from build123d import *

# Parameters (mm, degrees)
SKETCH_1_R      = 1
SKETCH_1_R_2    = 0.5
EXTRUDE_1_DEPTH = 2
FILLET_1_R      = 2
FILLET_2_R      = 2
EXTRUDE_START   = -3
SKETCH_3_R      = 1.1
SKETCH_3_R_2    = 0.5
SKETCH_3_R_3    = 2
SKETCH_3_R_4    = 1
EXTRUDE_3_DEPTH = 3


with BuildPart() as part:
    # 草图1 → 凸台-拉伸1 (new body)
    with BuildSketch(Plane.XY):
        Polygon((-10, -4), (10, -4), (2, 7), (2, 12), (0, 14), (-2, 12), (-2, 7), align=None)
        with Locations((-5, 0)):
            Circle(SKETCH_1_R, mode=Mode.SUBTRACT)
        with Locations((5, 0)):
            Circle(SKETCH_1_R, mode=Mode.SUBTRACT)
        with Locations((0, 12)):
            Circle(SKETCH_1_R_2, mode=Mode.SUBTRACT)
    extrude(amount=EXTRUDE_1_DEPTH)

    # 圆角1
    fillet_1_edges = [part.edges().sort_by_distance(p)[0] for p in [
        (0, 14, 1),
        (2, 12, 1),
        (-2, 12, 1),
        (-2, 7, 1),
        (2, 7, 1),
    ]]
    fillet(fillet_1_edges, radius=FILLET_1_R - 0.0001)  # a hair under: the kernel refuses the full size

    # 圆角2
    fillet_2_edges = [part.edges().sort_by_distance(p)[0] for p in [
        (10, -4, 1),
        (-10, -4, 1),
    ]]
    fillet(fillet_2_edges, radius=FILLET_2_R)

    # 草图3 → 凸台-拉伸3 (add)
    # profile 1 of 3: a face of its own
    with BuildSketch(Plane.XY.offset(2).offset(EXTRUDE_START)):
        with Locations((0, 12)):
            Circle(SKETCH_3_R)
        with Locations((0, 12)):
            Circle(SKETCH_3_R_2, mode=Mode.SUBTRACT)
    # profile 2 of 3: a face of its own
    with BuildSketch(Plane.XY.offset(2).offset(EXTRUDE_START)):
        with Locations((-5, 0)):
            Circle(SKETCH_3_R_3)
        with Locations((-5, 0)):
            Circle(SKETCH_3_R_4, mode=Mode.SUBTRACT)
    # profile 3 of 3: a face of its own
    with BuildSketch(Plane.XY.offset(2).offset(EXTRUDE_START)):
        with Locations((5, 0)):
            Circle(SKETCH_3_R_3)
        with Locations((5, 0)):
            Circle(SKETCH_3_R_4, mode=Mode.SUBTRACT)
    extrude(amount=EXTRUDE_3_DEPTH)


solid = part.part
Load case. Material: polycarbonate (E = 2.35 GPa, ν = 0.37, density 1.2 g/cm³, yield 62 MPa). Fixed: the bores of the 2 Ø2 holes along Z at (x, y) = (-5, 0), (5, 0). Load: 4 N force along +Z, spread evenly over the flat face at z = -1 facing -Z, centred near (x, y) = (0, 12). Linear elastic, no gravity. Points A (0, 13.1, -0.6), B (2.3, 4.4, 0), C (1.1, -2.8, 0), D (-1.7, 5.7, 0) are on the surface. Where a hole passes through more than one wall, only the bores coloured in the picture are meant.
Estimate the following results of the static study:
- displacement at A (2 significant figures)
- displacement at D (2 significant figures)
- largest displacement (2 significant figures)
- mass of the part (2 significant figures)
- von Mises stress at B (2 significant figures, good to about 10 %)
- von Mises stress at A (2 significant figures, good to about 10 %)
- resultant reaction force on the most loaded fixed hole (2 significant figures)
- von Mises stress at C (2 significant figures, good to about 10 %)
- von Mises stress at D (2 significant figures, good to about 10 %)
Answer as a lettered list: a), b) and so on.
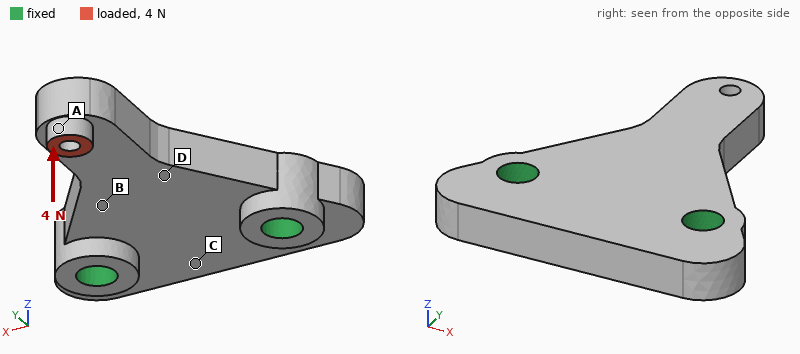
a) 0.23 mm
b) 0.046 mm
c) 0.23 mm
d) 0.37 g
e) 6.7 MPa
f) 1.3 MPa
g) 2.1 N
h) 0.66 MPa
i) 7.6 MPa
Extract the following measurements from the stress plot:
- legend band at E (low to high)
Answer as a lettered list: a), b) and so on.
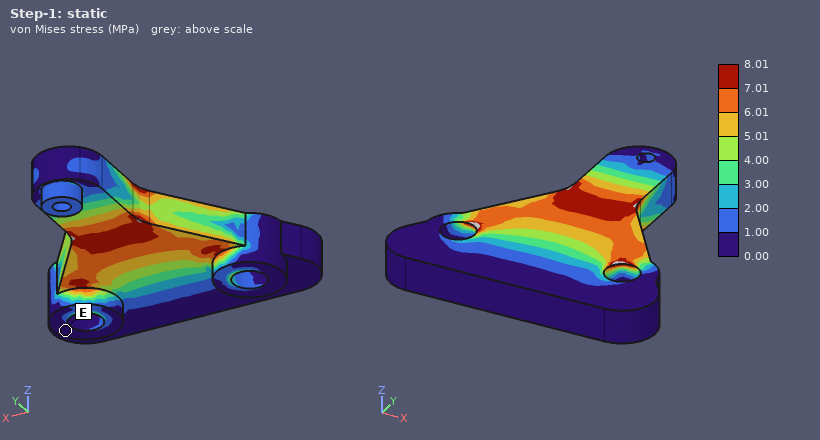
a) 0.00 to 1.00 MPa
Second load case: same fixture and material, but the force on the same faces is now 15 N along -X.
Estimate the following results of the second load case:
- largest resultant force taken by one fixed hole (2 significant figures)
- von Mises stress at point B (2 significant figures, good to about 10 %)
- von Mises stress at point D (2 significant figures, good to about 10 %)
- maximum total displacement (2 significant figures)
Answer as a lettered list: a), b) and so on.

a) 20 N
b) 6.6 MPa
c) 8.7 MPa
d) 0.18 mm
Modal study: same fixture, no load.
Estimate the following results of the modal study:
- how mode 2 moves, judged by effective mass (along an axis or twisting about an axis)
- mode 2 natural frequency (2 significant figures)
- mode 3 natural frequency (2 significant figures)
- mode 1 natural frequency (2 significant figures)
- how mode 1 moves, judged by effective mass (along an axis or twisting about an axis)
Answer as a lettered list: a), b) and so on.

a) along X
b) 12 kHz
c) 16 kHz
d) 3800 Hz
e) along Z
